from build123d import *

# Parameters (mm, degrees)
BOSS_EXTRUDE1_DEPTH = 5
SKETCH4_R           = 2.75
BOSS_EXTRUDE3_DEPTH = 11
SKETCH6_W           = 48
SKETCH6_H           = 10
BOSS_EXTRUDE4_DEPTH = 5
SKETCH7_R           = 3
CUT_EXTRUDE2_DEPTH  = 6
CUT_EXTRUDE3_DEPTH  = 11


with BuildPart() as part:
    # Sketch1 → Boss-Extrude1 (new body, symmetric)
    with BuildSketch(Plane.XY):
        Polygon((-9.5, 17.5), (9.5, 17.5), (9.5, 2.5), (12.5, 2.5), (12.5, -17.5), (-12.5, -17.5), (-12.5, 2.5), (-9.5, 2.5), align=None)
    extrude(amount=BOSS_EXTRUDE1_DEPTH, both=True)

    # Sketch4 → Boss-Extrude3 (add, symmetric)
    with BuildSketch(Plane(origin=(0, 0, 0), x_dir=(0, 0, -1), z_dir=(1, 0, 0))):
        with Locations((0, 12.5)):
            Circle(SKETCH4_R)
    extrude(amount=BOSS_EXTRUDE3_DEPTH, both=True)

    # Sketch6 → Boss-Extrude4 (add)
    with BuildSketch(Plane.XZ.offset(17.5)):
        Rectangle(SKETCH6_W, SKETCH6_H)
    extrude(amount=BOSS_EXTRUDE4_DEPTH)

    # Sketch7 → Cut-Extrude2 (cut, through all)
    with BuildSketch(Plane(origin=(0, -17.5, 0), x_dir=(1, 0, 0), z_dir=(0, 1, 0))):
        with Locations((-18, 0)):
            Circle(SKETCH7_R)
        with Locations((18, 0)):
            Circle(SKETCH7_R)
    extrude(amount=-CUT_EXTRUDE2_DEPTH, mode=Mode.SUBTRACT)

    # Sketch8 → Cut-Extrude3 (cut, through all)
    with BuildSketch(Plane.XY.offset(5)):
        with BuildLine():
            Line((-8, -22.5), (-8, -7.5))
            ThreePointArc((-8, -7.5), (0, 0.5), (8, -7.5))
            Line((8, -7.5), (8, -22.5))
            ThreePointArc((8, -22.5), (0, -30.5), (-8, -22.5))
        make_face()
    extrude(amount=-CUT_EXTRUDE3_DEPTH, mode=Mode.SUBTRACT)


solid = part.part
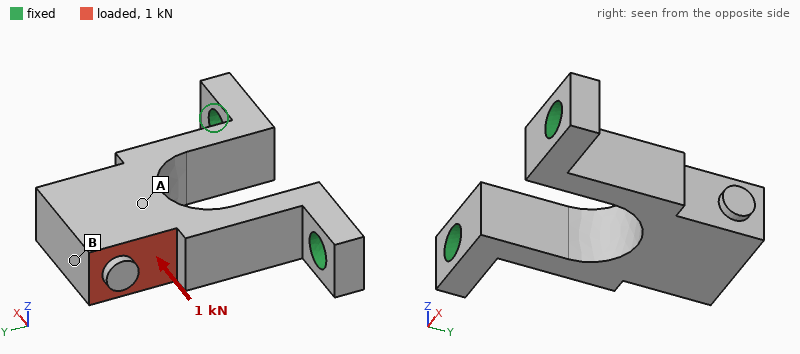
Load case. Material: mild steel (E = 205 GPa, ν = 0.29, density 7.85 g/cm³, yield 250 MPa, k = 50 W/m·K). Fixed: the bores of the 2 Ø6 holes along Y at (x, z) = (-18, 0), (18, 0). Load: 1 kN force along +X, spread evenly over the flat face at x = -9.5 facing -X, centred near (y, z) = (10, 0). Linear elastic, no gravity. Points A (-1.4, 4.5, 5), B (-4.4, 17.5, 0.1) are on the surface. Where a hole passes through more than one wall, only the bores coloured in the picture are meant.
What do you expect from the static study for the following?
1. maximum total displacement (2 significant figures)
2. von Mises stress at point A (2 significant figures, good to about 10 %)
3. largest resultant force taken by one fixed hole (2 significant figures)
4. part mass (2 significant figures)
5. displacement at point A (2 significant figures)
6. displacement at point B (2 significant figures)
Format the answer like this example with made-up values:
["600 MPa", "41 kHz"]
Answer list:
["23 µm", "23 MPa", "1.1 kN", "52 g", "21 µm", "23 µm"]
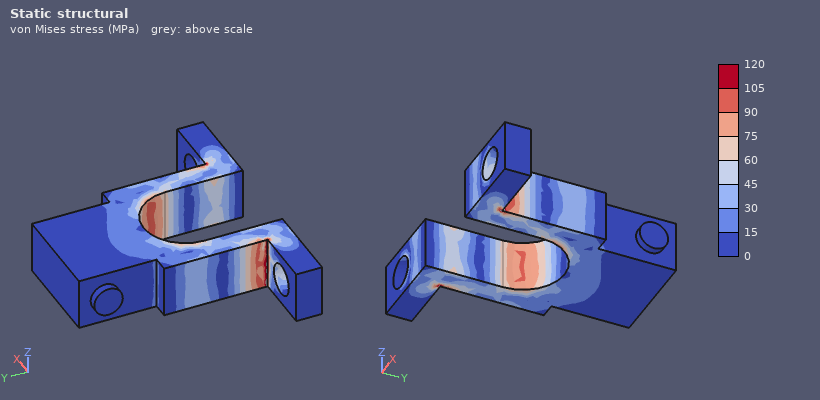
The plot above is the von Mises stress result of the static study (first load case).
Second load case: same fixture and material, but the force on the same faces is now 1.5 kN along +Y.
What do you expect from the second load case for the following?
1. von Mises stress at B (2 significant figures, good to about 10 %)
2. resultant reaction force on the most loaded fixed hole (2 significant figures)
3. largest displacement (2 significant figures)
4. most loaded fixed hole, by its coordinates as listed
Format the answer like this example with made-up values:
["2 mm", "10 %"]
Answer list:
["12 MPa", "1.4 kN", "11 µm", "(-18, 0)"]
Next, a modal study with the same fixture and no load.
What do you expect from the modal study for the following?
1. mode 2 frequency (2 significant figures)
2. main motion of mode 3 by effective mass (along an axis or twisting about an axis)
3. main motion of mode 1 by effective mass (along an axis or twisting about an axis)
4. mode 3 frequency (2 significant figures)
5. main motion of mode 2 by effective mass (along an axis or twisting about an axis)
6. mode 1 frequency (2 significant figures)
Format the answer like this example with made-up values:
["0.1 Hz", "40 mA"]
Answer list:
["5900 Hz", "twisting about Y", "along Z", "9800 Hz", "along X", "2600 Hz"]
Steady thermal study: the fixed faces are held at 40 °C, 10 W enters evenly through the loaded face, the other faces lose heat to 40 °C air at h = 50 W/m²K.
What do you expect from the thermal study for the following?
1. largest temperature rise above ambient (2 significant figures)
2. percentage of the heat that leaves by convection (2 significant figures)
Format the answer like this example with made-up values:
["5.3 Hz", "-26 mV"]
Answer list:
["50 K", "37 %"]
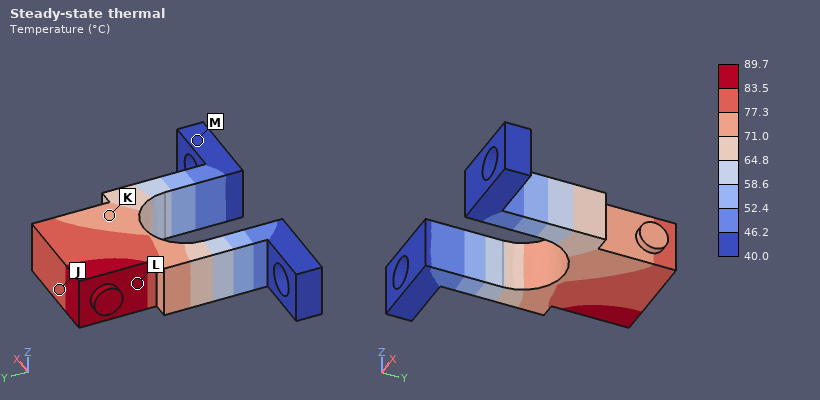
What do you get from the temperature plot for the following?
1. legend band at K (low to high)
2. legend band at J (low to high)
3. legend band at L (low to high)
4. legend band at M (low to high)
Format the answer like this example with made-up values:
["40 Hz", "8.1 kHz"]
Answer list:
["71.0 to 77.3 °C", "77.3 to 83.5 °C", "83.5 to 89.7 °C", "40.0 to 46.2 °C"]
